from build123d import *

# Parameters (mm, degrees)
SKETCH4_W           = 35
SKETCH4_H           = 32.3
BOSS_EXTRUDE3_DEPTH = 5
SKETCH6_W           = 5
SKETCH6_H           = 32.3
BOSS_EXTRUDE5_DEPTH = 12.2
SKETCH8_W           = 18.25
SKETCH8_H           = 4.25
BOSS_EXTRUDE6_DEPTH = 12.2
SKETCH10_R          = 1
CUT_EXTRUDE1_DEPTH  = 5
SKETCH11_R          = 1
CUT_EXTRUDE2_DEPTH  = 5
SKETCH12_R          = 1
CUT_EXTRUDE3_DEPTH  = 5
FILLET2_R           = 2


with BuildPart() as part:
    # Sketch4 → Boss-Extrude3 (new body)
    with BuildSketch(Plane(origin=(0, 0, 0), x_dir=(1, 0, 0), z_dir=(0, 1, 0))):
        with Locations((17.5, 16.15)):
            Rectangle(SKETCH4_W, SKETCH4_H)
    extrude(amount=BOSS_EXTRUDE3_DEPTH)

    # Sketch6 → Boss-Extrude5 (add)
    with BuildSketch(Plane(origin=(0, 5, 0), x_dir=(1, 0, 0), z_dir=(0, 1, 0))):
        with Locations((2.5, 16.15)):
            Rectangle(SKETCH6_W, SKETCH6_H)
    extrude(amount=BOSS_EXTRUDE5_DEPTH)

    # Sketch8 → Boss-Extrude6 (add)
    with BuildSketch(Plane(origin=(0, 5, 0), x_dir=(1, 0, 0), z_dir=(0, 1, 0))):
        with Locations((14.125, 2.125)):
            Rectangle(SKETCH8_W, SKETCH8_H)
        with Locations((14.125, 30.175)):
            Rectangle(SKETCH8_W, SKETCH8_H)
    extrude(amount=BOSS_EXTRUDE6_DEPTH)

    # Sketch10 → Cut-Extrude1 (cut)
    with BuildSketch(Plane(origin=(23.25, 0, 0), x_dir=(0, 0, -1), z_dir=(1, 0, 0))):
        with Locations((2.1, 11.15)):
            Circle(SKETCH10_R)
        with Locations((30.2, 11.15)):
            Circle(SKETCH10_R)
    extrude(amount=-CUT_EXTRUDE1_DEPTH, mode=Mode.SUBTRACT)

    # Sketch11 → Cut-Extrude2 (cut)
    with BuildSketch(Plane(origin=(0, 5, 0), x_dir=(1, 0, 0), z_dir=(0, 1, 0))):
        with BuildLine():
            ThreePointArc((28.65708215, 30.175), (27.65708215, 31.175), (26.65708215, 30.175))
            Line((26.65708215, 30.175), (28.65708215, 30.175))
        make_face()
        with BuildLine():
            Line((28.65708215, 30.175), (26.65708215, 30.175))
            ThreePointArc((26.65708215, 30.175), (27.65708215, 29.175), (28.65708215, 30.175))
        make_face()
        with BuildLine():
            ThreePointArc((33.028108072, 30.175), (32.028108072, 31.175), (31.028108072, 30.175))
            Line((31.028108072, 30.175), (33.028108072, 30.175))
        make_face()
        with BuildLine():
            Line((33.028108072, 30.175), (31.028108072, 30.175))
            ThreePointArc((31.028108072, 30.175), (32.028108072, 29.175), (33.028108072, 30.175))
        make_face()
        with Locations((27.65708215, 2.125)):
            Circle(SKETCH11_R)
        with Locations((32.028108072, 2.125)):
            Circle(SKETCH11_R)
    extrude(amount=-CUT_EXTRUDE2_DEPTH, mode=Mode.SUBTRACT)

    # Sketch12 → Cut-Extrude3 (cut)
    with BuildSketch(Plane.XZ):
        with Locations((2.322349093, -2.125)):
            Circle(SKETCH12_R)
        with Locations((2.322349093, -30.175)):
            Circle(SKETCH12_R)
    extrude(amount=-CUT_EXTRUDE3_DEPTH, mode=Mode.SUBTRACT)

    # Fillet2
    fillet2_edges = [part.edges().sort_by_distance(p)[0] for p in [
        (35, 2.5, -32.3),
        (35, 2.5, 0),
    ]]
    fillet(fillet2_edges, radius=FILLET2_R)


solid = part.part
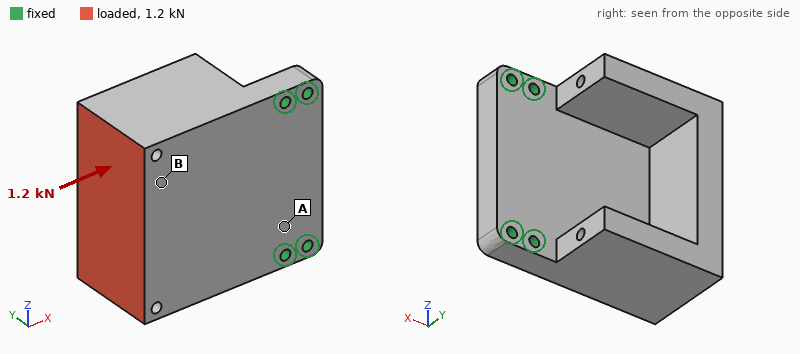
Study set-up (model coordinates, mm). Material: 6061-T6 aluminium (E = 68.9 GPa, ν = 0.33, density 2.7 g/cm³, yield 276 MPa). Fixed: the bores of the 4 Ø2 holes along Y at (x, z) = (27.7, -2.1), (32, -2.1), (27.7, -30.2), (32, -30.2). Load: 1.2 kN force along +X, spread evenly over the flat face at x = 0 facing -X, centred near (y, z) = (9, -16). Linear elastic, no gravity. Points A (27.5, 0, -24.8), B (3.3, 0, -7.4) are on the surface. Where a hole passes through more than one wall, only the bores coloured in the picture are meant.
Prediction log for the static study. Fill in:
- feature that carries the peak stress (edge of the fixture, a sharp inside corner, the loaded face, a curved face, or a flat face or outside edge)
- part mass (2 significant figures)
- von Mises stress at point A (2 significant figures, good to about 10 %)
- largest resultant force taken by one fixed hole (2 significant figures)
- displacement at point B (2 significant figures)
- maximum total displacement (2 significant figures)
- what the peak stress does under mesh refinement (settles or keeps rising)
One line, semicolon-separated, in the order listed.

edge of the fixture; 25 g; 33 MPa; 530 N; 0.081 mm; 0.12 mm; keeps rising
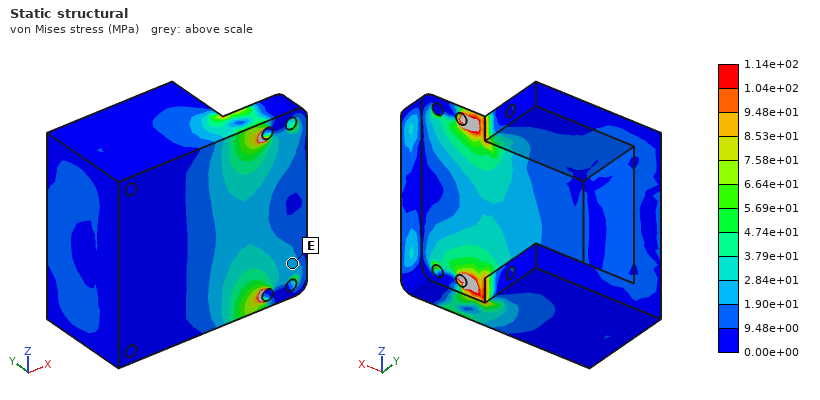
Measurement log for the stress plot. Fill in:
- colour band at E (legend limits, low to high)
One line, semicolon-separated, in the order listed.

1.90e+01 to 2.84e+01 MPa
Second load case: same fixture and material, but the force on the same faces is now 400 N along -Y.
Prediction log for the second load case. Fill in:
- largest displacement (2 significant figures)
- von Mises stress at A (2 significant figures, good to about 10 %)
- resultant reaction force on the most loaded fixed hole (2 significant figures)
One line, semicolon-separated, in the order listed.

0.15 mm; 53 MPa; 500 N
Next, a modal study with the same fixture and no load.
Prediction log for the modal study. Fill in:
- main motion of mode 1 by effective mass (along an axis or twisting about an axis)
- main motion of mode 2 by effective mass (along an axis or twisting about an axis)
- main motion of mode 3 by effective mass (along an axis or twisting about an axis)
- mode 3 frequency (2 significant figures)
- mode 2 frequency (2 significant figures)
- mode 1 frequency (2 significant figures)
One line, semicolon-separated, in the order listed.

along Y; along Z; along Z; 13 kHz; 6400 Hz; 2800 Hz
